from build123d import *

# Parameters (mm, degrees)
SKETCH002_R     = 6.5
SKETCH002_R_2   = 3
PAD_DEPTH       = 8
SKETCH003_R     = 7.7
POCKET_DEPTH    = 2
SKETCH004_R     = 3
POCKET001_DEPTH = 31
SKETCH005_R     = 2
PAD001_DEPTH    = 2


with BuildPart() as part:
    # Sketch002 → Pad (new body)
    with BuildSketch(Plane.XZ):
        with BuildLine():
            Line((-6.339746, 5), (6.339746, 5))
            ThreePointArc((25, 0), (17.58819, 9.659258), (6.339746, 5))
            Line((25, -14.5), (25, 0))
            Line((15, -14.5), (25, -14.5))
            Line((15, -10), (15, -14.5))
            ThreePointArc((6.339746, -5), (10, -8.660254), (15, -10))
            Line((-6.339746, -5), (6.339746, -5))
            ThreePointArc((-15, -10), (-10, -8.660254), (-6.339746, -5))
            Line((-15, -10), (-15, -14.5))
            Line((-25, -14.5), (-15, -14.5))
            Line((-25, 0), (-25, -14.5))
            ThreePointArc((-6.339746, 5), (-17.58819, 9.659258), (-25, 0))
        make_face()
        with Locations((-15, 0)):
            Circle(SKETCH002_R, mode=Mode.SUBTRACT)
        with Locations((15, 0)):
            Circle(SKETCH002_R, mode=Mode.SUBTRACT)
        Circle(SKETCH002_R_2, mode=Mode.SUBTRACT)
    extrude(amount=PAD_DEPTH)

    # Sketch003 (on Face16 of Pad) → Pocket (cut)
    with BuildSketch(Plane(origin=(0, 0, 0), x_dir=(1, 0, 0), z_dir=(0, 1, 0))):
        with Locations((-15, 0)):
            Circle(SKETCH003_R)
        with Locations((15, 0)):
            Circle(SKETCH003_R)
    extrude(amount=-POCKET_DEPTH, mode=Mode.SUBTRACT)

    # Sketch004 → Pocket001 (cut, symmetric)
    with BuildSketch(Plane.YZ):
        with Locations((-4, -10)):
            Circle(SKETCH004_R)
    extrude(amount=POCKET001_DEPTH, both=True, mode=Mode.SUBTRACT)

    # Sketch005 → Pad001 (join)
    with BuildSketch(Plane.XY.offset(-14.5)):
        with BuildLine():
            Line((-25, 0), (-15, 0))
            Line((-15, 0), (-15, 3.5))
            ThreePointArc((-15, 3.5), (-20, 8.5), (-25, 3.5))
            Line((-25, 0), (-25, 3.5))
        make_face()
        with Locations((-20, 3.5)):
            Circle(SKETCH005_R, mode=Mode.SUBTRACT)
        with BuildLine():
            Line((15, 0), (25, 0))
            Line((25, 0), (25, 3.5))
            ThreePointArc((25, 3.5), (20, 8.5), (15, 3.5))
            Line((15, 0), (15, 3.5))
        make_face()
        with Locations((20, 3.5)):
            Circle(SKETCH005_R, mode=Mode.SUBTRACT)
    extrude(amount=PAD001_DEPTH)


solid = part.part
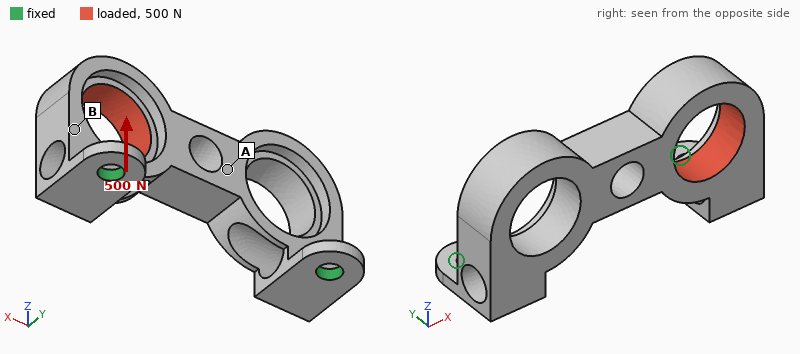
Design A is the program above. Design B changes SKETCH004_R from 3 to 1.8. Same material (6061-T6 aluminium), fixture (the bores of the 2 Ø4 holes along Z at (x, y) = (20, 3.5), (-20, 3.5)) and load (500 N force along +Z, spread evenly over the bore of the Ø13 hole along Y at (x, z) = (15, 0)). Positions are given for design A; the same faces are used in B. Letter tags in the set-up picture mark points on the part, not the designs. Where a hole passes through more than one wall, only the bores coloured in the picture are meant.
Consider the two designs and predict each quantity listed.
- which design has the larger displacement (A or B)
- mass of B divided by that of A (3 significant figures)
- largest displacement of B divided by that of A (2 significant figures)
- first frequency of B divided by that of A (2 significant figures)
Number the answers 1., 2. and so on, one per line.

1. A
2. 1.11
3. 0.83
4. 1.1
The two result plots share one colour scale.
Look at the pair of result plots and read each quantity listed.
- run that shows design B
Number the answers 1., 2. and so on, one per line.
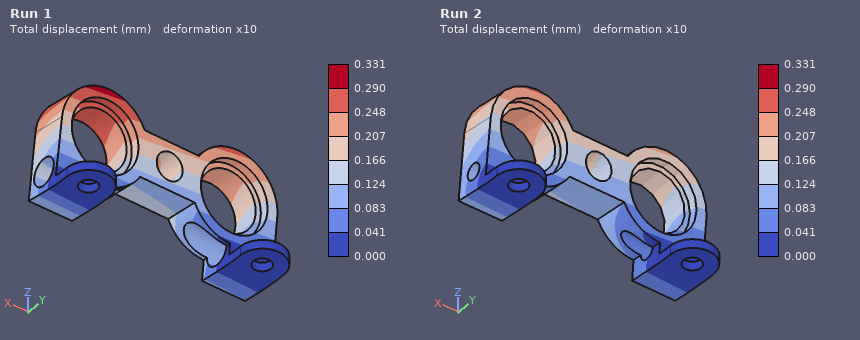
1. Run 2
